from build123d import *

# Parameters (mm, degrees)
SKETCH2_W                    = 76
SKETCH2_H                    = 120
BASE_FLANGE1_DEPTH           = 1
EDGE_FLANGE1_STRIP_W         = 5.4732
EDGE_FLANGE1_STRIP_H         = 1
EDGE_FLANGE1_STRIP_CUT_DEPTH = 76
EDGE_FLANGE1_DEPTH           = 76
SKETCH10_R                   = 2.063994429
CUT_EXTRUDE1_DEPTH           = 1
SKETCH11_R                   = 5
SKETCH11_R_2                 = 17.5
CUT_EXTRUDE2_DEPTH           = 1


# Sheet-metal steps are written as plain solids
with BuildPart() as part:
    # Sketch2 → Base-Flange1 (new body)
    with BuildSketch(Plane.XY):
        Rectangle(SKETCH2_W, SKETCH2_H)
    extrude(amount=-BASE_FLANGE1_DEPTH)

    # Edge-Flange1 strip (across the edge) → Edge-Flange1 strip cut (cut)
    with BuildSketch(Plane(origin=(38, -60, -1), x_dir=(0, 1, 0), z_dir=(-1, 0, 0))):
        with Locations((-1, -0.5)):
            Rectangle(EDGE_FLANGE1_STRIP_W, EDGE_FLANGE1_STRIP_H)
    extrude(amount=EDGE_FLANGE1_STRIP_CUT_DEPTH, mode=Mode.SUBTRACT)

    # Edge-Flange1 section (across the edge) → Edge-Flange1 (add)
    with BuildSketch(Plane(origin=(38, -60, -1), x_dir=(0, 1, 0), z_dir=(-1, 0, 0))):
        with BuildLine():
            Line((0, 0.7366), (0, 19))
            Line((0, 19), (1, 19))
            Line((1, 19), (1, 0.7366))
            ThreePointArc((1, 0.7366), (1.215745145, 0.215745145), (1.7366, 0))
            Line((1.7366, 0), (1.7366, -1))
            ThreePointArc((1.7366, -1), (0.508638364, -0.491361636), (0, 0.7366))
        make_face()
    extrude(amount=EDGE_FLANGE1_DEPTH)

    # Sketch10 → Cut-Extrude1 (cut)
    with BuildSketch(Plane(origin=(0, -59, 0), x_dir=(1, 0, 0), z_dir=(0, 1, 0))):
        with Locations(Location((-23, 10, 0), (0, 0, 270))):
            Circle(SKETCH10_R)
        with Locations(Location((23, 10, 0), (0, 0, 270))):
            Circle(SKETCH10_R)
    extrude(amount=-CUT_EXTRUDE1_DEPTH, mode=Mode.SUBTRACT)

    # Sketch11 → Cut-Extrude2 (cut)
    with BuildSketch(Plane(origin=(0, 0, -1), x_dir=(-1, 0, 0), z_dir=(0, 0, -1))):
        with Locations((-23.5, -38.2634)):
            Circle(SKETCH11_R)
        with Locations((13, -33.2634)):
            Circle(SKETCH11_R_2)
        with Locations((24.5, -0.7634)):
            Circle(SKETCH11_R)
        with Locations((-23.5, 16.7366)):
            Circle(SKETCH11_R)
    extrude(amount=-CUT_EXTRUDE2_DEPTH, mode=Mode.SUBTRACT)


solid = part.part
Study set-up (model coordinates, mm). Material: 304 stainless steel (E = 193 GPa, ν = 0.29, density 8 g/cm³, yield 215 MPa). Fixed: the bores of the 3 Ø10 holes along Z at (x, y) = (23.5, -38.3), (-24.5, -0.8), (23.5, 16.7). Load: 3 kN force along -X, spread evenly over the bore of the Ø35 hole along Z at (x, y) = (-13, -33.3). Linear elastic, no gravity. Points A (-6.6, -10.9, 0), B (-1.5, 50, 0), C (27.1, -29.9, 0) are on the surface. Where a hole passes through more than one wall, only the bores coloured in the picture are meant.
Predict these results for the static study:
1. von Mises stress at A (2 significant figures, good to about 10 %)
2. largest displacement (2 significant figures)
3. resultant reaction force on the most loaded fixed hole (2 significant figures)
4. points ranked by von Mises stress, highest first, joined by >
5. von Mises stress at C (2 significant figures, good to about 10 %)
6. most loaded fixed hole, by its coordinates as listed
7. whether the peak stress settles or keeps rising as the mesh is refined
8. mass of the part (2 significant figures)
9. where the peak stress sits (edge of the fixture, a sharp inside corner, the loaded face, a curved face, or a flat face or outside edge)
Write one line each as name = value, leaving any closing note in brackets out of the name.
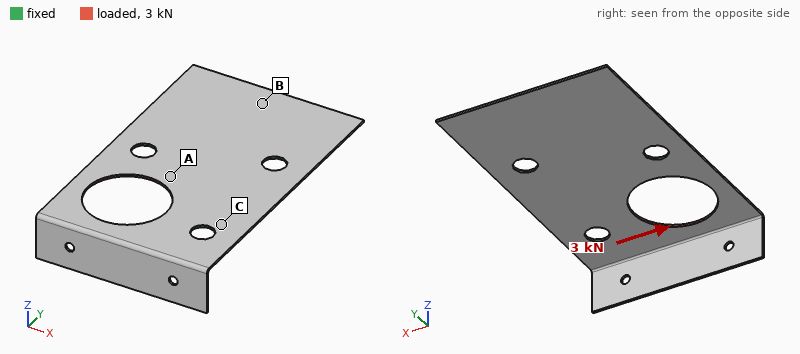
von Mises stress at A = 46 MPa
largest displacement = 44 µm
resultant reaction force on the most loaded fixed hole = 1.9 kN
points ranked by von Mises stress, highest first, joined by > = A > C > B
von Mises stress at C = 26 MPa
most loaded fixed hole, by its coordinates as listed = (23.5, -38.3)
whether the peak stress settles or keeps rising as the mesh is refined = keeps rising
mass of the part = 74 g
where the peak stress sits = edge of the fixture
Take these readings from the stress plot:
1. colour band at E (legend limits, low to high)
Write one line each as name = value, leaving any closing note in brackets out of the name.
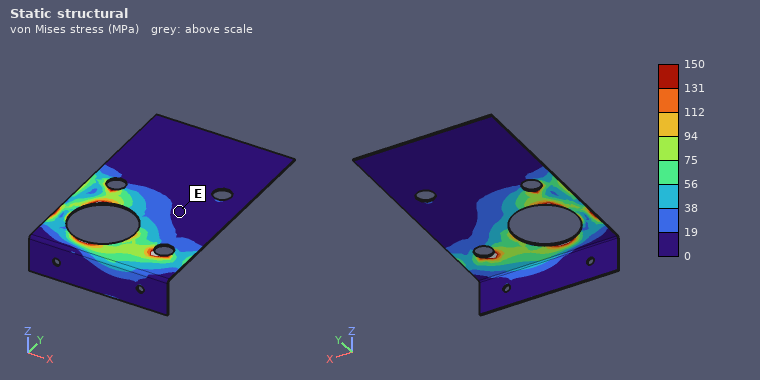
colour band at E = 0 to 19 MPa
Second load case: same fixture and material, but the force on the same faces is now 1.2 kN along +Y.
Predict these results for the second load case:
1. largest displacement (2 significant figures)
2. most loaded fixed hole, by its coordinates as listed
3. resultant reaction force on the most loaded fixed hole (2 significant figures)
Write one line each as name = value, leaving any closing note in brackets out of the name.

largest displacement = 15 µm
most loaded fixed hole, by its coordinates as listed = (-24.5, -0.8)
resultant reaction force on the most loaded fixed hole = 700 N
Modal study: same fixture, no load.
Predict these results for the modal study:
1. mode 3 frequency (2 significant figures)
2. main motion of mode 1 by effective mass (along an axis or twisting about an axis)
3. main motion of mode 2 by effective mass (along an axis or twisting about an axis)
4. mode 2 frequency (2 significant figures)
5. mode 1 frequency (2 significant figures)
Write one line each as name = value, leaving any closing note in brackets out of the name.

mode 3 frequency = 670 Hz
main motion of mode 1 by effective mass = along Z
main motion of mode 2 by effective mass = along Z
mode 2 frequency = 340 Hz
mode 1 frequency = 320 Hz
